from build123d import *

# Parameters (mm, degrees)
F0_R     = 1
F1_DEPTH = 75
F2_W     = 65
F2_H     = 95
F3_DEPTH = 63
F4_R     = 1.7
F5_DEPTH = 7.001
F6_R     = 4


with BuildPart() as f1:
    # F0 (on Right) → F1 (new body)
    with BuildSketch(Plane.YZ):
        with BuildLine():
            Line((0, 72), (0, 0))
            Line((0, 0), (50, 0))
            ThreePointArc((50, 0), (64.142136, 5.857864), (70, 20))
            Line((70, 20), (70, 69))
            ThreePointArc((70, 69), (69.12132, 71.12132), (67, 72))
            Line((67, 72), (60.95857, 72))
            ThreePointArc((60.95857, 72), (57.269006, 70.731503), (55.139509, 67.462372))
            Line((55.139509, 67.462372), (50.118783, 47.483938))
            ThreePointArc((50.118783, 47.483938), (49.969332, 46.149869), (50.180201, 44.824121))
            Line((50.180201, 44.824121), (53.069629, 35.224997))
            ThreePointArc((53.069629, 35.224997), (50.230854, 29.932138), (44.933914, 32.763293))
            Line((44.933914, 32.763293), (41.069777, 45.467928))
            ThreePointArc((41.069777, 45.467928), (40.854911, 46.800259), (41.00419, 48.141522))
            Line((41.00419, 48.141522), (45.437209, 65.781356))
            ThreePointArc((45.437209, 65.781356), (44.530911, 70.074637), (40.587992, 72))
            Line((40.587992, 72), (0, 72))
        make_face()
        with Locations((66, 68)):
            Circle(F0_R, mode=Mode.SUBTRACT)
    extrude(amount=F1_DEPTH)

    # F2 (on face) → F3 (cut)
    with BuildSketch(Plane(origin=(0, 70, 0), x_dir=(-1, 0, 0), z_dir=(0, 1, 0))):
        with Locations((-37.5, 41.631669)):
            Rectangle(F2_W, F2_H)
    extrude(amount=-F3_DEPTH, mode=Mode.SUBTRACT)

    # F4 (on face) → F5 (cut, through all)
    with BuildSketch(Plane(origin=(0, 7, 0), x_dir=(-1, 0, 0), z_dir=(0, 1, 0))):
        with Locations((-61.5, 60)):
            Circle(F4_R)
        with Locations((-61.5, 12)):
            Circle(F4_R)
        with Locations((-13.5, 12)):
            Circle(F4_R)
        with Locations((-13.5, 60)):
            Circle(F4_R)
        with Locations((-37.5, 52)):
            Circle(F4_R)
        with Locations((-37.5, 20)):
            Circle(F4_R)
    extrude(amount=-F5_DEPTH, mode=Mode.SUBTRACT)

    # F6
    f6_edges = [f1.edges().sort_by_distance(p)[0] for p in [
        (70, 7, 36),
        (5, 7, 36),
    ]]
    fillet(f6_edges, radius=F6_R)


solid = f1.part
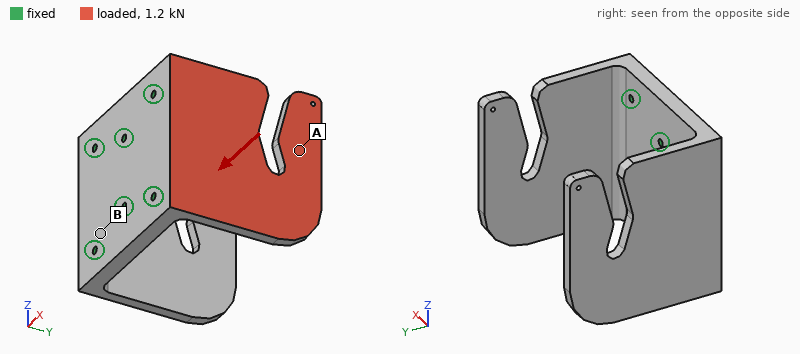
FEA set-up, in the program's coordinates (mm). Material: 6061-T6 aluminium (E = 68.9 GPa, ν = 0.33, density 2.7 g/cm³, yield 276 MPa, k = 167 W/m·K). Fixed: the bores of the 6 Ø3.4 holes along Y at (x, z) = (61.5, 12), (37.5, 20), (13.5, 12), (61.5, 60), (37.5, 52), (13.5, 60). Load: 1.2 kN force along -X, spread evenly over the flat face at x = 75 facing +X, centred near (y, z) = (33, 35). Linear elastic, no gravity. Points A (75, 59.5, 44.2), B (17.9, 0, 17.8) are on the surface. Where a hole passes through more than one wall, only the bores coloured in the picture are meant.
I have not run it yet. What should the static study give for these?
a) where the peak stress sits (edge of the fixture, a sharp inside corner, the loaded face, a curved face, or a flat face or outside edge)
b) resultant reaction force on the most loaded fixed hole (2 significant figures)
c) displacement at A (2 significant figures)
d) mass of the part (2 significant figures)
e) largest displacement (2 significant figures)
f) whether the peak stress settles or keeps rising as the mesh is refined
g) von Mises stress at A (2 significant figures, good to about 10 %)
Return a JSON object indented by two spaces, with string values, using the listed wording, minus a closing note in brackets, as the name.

{
  "where the peak stress sits": "edge of the fixture",
  "resultant reaction force on the most loaded fixed hole": "550 N",
  "displacement at A": "0.87 mm",
  "mass of the part": "210 g",
  "largest displacement": "1.3 mm",
  "whether the peak stress settles or keeps rising as the mesh is refined": "keeps rising",
  "von Mises stress at A": "20 MPa"
}
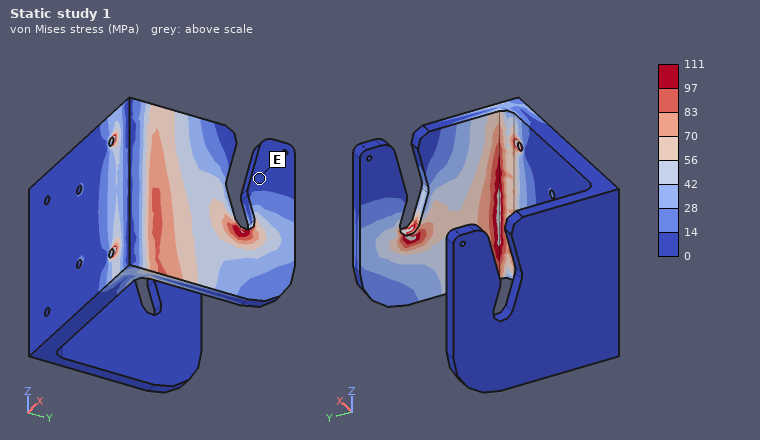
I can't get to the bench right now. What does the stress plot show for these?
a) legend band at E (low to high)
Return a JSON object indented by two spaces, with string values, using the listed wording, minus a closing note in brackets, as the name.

{
  "legend band at E": "0 to 14 MPa"
}
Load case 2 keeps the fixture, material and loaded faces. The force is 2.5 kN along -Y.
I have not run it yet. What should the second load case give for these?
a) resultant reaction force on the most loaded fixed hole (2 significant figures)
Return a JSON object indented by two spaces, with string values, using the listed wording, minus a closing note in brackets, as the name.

{
  "resultant reaction force on the most loaded fixed hole": "1.6 kN"
}
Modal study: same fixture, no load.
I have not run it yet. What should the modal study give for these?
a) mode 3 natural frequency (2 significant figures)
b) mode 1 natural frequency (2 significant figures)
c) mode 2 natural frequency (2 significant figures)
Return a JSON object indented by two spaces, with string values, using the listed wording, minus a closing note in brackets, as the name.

{
  "mode 3 natural frequency": "1600 Hz",
  "mode 1 natural frequency": "820 Hz",
  "mode 2 natural frequency": "820 Hz"
}
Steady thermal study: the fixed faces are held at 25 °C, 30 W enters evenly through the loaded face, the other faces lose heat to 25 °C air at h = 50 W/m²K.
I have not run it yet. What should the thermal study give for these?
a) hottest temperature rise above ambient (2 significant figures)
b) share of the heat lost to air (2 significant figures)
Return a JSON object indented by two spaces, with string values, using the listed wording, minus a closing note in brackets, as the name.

{
  "hottest temperature rise above ambient": "25 K",
  "share of the heat lost to air": "15 %"
}
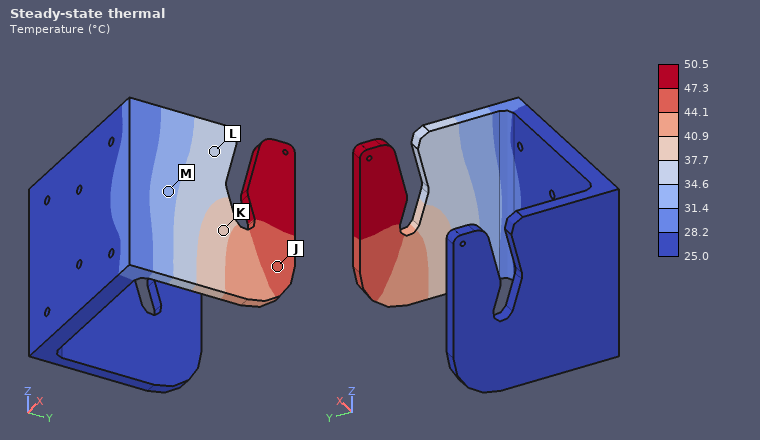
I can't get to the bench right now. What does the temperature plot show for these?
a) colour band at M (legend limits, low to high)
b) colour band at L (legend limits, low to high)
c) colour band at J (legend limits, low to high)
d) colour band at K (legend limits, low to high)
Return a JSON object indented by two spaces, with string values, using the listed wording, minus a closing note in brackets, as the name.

{
  "colour band at M": "31.4 to 34.6 °C",
  "colour band at L": "34.6 to 37.7 °C",
  "colour band at J": "44.1 to 47.3 °C",
  "colour band at K": "37.7 to 40.9 °C"
}
